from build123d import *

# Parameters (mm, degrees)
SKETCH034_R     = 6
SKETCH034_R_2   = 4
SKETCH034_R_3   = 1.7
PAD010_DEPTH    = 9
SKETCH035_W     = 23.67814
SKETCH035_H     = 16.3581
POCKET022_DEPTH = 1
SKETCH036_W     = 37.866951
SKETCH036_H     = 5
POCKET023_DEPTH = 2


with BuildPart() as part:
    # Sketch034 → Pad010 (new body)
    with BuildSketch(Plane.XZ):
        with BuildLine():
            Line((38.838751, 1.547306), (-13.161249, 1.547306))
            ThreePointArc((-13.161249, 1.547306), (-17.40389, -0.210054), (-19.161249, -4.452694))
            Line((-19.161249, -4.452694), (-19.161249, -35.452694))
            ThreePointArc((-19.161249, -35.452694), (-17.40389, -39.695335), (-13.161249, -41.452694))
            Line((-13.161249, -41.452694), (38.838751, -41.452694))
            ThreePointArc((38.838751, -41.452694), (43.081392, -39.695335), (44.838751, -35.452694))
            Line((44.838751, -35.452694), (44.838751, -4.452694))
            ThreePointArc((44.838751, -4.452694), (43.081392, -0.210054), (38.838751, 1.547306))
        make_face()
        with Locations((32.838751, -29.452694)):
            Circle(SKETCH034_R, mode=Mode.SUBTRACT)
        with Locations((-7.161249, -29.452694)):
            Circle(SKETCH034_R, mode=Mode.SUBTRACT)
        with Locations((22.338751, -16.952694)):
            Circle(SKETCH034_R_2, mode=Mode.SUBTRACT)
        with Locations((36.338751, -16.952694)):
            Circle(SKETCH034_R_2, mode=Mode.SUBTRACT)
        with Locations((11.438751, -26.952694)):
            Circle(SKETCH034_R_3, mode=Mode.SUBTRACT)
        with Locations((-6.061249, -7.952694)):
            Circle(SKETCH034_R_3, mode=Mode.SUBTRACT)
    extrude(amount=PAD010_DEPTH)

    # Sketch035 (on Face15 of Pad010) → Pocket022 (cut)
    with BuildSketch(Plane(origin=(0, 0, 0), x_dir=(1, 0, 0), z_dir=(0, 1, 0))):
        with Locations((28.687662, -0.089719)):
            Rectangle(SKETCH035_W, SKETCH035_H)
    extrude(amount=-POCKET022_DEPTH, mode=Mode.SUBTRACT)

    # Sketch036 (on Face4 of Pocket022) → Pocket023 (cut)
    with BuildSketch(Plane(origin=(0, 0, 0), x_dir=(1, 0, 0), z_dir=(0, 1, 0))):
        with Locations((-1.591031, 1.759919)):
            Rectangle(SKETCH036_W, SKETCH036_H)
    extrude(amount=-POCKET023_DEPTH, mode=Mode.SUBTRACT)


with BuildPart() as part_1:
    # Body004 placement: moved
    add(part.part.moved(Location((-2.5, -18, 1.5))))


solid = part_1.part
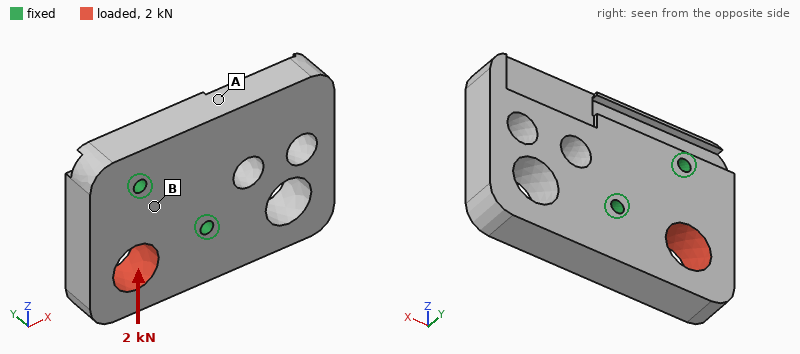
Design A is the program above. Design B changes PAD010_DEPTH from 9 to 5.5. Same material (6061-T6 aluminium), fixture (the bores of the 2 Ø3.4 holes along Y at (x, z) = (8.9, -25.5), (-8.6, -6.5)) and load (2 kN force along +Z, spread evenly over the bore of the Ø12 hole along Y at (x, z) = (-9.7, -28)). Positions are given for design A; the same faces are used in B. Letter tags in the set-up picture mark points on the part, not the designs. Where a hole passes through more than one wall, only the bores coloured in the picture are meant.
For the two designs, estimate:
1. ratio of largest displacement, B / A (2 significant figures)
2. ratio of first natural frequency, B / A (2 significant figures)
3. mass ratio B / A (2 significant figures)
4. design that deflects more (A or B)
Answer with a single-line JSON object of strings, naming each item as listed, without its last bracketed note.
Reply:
{"ratio of largest displacement, B / A": "1.6", "ratio of first natural frequency, B / A": "0.67", "mass ratio B / A": "0.60", "design that deflects more": "B"}
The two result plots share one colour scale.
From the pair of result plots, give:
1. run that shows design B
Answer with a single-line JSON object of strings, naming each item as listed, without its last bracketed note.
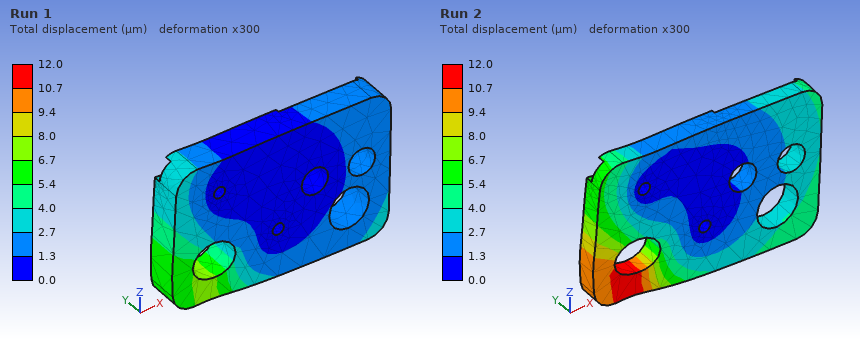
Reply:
{"run that shows design B": "Run 2"}
